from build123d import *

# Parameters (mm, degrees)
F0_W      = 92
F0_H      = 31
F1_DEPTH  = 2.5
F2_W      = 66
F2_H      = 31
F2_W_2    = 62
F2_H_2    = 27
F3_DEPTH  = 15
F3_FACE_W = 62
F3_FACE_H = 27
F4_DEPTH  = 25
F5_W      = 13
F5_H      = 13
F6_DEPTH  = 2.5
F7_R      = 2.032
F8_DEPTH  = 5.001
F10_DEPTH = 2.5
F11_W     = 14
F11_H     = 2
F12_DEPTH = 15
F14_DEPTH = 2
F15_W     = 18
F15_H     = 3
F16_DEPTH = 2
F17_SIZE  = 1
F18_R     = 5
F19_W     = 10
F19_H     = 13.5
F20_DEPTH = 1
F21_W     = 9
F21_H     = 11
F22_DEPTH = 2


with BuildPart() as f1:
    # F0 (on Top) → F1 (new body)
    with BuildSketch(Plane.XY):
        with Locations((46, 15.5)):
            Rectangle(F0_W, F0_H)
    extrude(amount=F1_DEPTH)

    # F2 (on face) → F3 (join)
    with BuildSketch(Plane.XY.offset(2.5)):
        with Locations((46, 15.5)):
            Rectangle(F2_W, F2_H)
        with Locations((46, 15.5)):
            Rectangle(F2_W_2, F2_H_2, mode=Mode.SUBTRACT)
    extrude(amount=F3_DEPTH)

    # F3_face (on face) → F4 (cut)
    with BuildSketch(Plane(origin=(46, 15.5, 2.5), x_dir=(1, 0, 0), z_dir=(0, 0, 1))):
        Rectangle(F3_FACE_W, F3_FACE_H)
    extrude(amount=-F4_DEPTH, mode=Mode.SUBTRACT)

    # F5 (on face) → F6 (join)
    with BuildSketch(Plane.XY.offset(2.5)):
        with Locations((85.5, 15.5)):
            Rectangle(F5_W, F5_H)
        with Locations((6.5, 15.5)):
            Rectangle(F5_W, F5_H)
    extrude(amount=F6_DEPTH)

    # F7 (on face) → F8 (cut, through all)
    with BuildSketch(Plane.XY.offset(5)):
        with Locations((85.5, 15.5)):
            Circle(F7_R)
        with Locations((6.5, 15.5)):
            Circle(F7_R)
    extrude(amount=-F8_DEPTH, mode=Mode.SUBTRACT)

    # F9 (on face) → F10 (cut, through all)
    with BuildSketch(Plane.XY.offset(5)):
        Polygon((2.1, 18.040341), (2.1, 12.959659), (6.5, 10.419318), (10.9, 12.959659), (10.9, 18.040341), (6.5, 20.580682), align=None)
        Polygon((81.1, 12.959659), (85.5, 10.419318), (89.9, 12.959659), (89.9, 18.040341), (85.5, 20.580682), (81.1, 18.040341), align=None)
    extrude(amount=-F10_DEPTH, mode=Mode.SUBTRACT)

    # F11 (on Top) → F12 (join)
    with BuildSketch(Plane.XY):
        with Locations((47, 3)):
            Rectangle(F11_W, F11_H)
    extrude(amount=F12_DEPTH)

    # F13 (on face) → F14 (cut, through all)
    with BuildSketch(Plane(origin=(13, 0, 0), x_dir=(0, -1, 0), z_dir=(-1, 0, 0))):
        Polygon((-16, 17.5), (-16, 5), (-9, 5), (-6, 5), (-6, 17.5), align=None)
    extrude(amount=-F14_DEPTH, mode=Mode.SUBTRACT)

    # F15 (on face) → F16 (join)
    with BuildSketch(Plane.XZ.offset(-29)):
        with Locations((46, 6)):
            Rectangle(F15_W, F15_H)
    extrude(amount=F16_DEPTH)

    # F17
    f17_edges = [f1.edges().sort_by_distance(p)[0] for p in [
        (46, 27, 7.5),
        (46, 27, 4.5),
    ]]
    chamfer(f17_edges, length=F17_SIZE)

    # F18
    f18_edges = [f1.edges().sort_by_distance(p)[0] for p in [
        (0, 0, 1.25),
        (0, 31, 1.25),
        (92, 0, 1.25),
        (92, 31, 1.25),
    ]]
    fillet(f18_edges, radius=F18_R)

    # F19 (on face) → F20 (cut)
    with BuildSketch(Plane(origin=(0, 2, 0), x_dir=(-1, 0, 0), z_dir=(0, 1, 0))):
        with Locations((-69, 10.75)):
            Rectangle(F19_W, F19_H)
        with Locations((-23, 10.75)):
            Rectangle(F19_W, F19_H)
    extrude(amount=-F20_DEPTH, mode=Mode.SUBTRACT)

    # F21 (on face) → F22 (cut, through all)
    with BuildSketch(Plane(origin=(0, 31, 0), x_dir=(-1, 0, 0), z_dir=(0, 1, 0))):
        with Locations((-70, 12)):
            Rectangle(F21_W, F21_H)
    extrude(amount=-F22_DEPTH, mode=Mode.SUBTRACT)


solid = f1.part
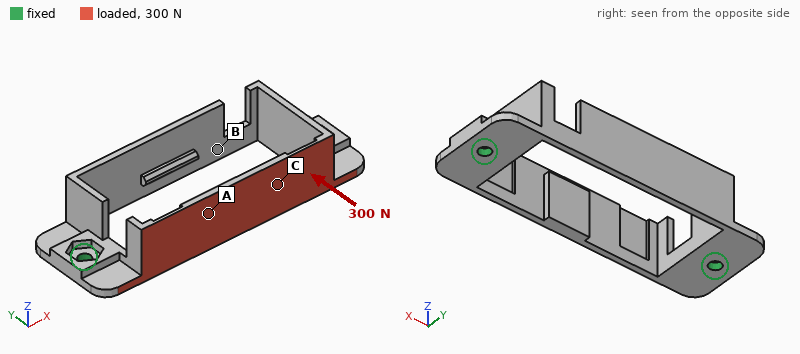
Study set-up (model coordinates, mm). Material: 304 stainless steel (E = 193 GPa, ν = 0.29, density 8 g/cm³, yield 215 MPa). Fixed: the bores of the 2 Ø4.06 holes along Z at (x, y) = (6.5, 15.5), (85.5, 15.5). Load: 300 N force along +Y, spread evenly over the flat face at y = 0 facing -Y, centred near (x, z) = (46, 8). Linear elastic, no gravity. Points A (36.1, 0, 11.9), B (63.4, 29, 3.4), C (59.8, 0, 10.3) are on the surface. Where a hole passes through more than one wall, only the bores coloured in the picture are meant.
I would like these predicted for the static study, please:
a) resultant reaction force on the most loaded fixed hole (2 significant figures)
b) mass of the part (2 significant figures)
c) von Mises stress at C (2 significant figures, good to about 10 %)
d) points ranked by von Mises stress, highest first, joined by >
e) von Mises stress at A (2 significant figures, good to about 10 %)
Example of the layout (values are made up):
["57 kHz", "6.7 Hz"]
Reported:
["160 N", "70 g", "53 MPa", "A > C > B", "69 MPa"]
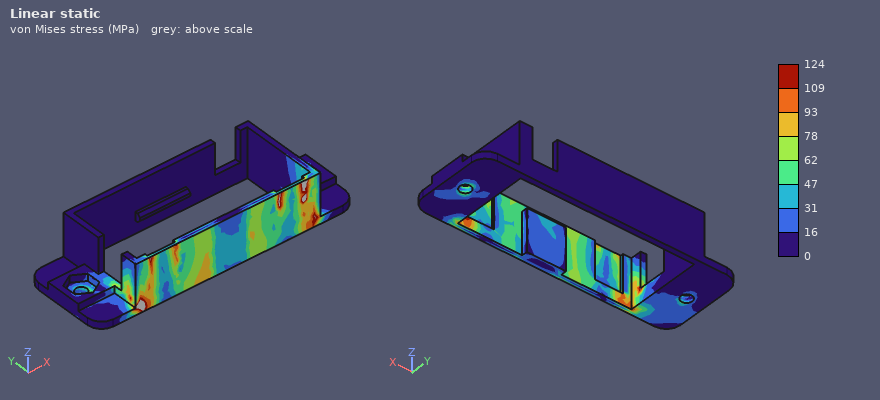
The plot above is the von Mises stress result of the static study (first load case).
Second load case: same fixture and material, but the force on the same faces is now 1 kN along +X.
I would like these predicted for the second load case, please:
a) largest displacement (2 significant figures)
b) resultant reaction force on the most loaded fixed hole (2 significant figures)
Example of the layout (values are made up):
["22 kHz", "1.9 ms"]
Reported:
["31 µm", "520 N"]
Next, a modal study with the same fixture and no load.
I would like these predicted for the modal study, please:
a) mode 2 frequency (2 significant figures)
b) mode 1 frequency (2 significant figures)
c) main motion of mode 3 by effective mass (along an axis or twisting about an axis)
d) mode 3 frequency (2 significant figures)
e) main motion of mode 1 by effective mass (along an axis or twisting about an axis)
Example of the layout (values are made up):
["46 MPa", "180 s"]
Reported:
["2000 Hz", "1800 Hz", "twisting about X", "3100 Hz", "along Y"]
